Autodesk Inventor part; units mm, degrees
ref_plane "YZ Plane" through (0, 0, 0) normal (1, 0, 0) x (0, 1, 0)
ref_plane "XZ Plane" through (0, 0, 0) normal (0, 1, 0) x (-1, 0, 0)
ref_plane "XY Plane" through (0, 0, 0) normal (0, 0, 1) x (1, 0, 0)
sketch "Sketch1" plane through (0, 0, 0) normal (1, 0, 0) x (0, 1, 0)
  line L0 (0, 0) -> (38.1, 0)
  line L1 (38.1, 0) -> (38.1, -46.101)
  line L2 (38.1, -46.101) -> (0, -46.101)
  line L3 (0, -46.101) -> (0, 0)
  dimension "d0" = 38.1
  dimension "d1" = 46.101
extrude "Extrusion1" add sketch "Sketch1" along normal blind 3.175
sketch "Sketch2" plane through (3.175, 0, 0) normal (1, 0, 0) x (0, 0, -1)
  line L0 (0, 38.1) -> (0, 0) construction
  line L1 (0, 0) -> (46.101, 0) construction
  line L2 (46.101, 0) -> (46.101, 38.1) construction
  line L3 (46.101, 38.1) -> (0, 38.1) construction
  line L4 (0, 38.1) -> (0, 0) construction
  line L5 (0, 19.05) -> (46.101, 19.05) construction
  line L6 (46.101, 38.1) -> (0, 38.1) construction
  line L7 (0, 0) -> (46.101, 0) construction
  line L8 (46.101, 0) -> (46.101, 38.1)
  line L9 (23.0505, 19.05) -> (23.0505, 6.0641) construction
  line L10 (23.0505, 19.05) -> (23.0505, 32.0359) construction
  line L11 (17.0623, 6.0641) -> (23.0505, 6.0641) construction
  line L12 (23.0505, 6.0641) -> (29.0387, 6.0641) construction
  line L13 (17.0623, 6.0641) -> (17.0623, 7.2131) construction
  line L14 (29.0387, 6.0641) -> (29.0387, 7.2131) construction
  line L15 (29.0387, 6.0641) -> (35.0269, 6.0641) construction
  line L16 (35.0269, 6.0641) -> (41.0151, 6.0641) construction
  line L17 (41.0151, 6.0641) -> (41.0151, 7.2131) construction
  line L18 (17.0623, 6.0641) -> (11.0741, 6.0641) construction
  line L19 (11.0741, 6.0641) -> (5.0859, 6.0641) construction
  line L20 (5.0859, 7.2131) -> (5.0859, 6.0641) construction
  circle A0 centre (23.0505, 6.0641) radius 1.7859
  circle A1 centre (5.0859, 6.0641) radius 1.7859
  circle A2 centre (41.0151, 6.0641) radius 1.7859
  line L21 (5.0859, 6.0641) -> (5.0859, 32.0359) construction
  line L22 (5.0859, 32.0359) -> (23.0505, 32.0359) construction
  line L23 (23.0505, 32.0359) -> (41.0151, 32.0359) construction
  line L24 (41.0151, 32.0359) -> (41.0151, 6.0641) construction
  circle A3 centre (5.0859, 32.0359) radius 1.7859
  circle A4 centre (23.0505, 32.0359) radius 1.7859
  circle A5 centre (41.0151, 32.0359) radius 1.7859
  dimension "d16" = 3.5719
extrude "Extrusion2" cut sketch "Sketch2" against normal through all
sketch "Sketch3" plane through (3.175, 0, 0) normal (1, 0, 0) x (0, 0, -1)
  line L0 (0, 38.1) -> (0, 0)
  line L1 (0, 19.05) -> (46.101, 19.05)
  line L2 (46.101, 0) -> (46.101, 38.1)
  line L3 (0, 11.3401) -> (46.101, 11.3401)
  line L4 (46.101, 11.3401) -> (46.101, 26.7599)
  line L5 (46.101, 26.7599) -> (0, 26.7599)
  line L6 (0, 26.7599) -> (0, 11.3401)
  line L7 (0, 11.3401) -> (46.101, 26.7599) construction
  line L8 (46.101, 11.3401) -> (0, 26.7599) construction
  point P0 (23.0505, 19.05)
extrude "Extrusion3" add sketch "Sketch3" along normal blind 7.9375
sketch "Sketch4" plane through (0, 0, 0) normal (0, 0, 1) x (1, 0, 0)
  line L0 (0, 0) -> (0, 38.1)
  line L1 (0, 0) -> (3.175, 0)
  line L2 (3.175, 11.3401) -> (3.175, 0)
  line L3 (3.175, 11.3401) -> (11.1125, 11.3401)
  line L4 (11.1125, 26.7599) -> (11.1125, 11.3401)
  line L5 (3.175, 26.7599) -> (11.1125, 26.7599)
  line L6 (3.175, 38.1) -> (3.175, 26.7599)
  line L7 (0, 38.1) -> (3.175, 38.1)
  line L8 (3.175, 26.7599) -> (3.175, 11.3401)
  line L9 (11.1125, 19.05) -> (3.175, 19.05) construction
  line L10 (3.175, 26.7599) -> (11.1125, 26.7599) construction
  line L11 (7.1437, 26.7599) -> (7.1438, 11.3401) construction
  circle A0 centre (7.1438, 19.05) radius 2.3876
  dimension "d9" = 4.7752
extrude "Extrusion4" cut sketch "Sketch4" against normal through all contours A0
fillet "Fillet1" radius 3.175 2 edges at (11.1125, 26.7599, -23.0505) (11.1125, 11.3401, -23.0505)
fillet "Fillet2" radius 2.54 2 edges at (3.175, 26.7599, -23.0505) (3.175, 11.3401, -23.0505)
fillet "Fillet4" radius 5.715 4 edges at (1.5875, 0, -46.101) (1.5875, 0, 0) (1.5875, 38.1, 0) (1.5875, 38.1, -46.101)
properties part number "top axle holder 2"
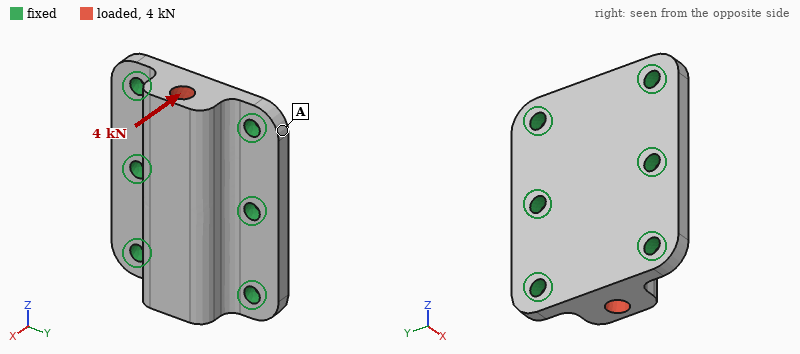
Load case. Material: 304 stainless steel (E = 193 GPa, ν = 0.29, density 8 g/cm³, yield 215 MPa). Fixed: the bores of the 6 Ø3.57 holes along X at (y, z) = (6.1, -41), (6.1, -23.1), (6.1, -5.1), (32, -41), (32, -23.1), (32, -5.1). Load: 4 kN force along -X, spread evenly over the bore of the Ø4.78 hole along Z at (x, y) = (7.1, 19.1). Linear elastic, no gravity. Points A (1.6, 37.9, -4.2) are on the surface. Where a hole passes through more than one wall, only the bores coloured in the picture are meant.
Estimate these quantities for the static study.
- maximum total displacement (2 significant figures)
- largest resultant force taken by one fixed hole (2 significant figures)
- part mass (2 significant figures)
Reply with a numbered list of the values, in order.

1. 3.8 µm
2. 840 N
3. 80 g
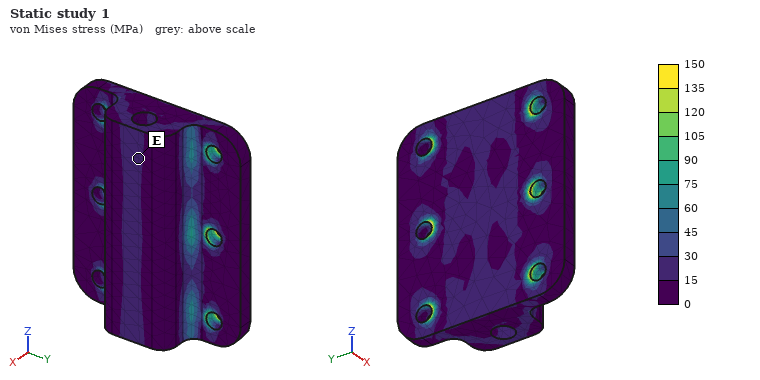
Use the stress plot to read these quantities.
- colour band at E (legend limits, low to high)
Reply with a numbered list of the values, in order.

1. 15 to 30 MPa
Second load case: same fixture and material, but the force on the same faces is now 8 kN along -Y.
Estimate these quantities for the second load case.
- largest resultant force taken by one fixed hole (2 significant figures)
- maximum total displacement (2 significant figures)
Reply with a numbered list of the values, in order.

1. 1.7 kN
2. 4.6 µm
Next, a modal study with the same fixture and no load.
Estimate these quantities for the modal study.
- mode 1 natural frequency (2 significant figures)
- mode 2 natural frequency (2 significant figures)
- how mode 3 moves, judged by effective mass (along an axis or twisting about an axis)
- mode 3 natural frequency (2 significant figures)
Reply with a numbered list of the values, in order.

1. 23 kHz
2. 23 kHz
3. along Y
4. 35 kHz
